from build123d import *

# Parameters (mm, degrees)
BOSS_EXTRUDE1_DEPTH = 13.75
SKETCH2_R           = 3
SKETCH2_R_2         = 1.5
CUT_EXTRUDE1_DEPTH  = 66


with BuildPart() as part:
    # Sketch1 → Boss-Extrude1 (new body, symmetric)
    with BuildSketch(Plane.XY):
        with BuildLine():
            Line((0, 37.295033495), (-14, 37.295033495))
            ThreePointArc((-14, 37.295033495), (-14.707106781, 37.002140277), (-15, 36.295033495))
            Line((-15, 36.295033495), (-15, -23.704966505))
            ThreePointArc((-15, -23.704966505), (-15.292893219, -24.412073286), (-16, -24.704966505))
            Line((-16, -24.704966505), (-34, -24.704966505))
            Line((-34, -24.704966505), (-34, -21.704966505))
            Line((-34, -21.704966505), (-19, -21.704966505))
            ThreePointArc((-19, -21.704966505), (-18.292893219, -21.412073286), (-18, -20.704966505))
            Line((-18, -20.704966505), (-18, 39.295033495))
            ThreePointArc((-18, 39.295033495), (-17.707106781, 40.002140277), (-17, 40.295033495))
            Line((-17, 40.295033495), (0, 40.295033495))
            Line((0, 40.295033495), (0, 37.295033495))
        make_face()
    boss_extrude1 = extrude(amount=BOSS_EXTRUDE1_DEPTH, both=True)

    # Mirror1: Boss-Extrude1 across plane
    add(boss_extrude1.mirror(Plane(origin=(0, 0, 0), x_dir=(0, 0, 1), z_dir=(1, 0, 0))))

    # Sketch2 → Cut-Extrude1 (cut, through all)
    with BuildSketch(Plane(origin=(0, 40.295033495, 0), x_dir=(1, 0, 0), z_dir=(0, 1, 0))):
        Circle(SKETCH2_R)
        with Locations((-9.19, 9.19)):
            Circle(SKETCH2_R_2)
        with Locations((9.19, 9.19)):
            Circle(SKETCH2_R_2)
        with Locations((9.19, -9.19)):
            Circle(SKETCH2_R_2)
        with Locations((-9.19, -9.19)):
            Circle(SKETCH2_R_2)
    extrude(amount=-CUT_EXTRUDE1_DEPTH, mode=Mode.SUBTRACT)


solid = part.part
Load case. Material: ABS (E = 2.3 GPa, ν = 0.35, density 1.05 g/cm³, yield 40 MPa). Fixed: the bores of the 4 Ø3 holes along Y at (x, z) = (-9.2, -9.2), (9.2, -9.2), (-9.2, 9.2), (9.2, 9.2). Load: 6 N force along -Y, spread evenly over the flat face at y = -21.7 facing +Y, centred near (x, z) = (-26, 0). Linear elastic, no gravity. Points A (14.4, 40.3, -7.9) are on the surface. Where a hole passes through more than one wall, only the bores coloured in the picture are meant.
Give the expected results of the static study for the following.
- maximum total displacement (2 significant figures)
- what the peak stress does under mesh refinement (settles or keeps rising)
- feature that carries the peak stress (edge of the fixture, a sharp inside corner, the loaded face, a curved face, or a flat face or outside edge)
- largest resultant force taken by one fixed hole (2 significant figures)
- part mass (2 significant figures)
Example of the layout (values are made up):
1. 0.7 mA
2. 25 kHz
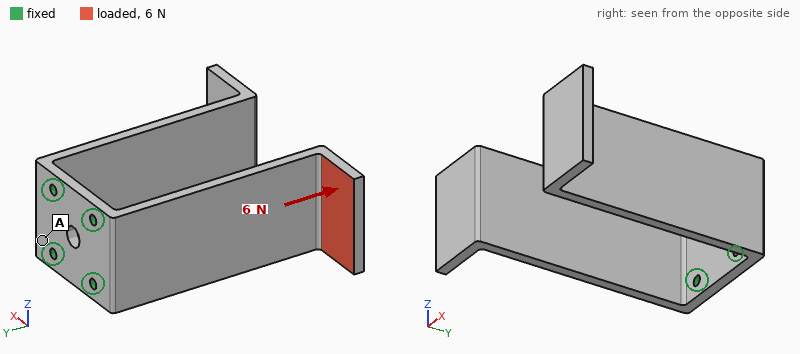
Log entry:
1. 1.2 mm
2. keeps rising
3. edge of the fixture
4. 3.6 N
5. 16 g
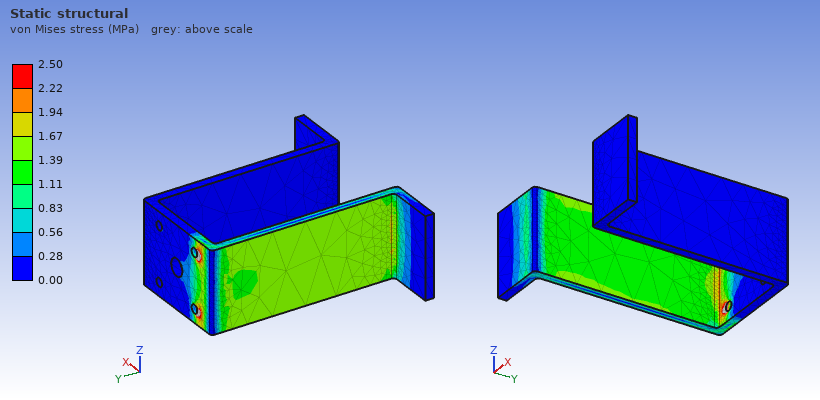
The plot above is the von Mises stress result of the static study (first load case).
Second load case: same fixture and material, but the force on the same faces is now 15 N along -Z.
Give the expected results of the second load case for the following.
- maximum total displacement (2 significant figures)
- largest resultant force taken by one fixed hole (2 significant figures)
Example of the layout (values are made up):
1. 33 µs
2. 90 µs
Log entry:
1. 1.1 mm
2. 49 N
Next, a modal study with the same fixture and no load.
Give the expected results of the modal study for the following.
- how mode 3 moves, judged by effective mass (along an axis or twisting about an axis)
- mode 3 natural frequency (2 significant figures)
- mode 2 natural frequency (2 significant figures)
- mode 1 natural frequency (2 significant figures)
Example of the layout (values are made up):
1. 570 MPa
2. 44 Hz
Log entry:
1. along Z
2. 470 Hz
3. 110 Hz
4. 110 Hz
